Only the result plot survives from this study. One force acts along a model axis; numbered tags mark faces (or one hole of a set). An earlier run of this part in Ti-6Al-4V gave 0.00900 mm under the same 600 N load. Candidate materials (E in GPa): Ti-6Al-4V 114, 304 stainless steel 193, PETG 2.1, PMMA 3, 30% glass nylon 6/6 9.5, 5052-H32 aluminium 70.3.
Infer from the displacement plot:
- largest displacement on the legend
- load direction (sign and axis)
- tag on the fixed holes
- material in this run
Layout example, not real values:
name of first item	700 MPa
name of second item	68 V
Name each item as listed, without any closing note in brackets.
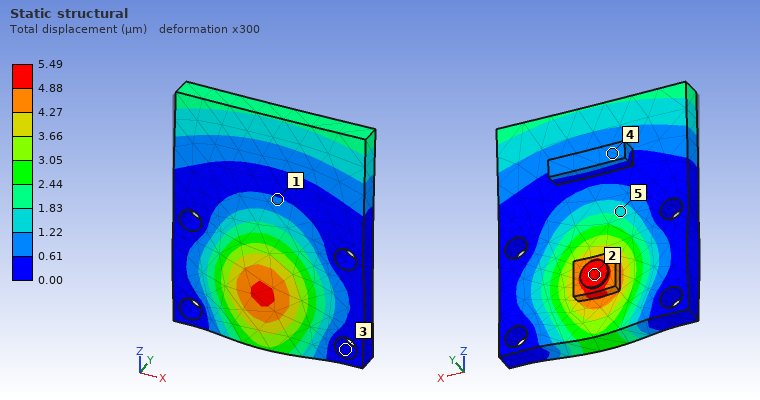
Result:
largest displacement on the legend	5.49 µm
load direction	-Y
tag on the fixed holes	3
material in this run	304 stainless steel
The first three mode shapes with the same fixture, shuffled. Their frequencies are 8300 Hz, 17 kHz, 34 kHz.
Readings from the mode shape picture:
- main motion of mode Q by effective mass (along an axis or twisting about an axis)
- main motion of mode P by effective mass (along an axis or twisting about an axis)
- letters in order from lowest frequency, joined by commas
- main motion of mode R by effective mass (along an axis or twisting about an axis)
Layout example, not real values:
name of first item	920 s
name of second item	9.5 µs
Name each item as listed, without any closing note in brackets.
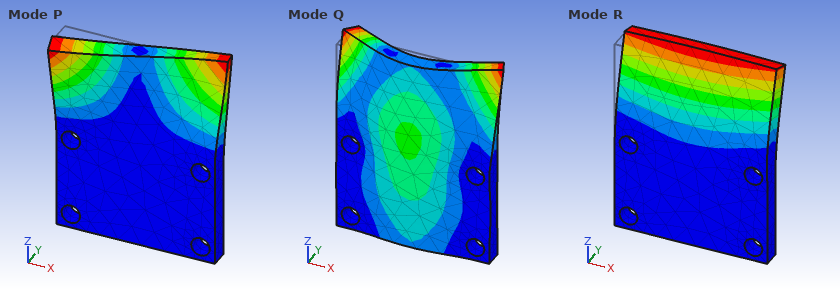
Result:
main motion of mode Q by effective mass	along Y
main motion of mode P by effective mass	twisting about Z
letters in order from lowest frequency, joined by commas	R, P, Q
main motion of mode R by effective mass	along Y
